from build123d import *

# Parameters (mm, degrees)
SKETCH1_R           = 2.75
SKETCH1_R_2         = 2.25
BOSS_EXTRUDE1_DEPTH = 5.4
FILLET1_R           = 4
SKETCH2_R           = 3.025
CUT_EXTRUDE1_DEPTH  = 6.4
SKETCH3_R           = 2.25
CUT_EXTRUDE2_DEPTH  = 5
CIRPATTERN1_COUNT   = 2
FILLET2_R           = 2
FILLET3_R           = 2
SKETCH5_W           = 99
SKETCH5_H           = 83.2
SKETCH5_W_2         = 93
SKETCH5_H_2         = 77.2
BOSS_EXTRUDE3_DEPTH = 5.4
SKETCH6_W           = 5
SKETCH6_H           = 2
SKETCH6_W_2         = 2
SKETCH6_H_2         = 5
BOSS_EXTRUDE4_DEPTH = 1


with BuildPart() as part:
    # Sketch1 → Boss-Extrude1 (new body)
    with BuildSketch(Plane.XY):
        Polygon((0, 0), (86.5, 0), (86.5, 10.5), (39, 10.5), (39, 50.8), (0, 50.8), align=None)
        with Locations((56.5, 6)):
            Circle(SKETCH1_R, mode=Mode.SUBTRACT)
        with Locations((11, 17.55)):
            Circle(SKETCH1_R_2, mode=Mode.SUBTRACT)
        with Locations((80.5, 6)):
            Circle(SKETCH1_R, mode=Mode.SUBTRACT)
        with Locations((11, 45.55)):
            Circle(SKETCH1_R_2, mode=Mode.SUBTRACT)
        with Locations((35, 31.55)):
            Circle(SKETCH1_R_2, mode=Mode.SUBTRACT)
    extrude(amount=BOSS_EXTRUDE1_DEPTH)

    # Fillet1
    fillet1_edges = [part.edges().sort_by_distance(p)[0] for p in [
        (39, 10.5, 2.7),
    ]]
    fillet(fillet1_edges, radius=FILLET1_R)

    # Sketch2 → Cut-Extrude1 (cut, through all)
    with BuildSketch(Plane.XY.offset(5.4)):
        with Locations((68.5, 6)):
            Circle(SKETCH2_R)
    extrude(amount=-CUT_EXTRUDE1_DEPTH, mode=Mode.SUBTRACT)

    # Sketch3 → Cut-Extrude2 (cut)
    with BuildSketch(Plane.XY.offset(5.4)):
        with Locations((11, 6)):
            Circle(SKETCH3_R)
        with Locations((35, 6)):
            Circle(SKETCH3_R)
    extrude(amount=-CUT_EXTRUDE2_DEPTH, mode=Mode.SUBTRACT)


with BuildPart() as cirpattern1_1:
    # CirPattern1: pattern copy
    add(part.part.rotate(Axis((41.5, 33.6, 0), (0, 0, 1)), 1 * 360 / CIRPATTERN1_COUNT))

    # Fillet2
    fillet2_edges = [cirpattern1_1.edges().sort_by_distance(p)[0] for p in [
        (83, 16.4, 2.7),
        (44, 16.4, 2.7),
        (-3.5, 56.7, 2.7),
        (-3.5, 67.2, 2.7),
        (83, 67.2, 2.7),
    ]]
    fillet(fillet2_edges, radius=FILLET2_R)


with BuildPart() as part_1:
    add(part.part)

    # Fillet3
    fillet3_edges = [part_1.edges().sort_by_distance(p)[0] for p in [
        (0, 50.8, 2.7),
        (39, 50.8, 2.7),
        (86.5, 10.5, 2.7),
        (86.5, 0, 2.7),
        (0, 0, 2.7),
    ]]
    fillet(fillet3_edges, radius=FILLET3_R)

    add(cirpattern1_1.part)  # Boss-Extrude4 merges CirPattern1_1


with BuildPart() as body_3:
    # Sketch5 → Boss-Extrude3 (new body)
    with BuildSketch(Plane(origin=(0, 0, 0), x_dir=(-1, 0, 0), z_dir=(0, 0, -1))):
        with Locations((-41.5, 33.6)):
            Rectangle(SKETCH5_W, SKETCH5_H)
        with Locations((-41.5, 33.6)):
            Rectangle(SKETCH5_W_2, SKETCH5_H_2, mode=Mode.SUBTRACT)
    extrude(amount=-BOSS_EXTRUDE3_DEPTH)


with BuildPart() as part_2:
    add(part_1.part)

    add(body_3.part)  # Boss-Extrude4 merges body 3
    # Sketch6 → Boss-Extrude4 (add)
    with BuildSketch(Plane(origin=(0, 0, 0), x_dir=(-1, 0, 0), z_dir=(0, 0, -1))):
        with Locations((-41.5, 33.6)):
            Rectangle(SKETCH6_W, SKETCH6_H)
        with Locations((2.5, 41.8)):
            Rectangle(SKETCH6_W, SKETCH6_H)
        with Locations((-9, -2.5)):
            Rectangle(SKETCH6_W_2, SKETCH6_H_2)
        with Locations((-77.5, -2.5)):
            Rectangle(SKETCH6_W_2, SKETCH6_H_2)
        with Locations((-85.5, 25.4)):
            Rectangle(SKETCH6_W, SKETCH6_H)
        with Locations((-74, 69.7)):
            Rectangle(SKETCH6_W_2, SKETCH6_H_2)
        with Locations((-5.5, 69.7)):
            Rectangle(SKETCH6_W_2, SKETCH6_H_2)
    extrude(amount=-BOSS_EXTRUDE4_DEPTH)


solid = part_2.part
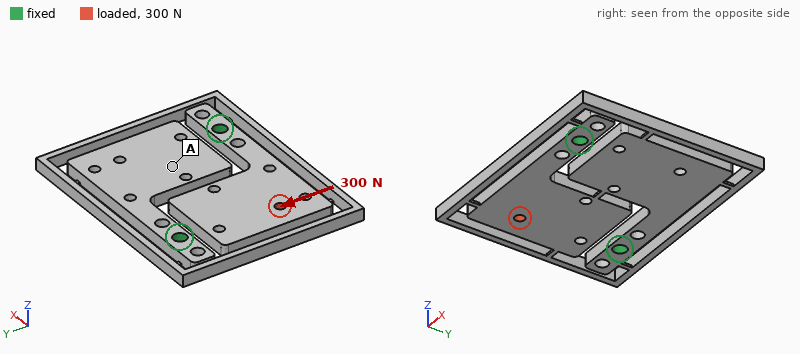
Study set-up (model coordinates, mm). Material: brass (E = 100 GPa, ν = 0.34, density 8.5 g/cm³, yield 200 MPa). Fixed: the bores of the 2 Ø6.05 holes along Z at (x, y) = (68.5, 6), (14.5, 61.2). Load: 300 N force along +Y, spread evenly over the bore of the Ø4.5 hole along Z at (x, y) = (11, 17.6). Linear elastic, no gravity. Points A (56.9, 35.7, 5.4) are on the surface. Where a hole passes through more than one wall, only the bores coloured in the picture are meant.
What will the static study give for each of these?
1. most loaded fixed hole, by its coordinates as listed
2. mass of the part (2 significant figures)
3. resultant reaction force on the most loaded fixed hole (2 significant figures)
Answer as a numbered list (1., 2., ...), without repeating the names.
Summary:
1. (68.5, 6)
2. 260 g
3. 280 N
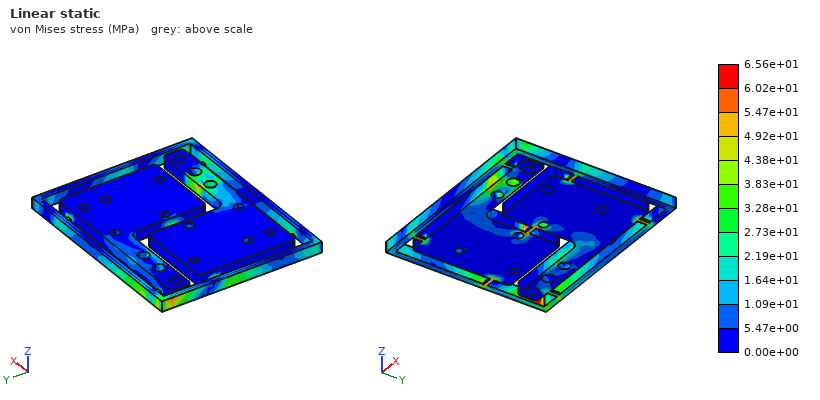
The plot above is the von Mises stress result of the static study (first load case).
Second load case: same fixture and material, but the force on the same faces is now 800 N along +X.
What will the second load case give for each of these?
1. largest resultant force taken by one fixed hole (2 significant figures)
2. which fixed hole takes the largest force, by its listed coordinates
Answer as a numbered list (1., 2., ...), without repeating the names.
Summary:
1. 640 N
2. (68.5, 6)
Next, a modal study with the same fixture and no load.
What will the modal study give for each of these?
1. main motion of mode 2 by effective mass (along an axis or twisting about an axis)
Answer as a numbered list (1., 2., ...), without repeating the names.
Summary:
1. along Z
